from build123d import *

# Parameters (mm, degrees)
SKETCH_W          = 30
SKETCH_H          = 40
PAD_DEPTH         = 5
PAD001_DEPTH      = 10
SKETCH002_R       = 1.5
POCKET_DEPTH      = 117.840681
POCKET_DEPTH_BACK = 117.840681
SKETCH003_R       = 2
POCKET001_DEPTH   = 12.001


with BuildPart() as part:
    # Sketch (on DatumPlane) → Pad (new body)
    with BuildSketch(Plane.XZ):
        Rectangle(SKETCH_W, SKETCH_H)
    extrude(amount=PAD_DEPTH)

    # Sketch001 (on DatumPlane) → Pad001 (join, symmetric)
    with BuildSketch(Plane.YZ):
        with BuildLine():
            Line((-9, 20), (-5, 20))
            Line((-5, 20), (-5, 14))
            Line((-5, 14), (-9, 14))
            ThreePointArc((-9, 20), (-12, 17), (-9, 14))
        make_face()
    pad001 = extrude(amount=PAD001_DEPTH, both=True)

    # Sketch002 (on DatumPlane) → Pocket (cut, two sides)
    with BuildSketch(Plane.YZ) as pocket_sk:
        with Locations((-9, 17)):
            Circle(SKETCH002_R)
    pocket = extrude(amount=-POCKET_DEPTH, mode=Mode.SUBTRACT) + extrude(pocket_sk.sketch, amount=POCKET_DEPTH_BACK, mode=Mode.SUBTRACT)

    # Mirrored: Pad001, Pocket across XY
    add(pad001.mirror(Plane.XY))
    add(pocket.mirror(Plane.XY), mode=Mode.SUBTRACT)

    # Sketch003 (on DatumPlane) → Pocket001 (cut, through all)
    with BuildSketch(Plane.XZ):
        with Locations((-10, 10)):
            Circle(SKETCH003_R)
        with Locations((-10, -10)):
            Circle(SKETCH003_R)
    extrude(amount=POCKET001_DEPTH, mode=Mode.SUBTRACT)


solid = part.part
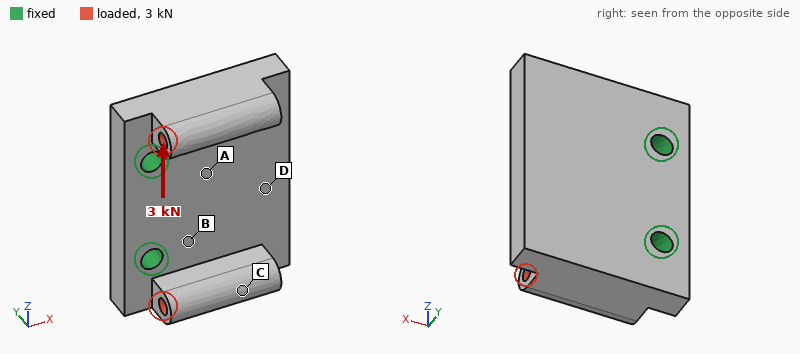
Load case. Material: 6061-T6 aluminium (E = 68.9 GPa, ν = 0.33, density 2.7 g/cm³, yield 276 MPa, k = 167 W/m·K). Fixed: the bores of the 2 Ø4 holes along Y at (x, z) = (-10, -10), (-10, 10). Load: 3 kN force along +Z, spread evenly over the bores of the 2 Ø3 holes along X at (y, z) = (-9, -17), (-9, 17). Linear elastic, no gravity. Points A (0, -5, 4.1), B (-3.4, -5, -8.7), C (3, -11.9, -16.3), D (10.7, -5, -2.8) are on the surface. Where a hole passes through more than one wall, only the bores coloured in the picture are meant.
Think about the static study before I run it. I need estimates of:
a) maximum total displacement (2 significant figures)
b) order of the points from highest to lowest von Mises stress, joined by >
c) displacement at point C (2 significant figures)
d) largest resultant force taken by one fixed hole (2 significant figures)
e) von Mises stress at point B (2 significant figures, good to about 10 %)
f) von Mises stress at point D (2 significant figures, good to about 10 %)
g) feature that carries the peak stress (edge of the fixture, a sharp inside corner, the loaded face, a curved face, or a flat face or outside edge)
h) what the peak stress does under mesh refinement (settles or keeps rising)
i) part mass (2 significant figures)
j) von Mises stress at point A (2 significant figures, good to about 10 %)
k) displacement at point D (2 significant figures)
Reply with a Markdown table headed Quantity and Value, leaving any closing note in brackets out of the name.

| Quantity | Value |
|---|---|
| maximum total displacement | 84 µm |
| order of the points from highest to lowest von Mises stress, joined by > | B > A > D > C |
| displacement at point C | 69 µm |
| largest resultant force taken by one fixed hole | 2.0 kN |
| von Mises stress at point B | 75 MPa |
| von Mises stress at point D | 27 MPa |
| feature that carries the peak stress | edge of the fixture |
| what the peak stress does under mesh refinement | keeps rising |
| part mass | 19 g |
| von Mises stress at point A | 52 MPa |
| displacement at point D | 18 µm |
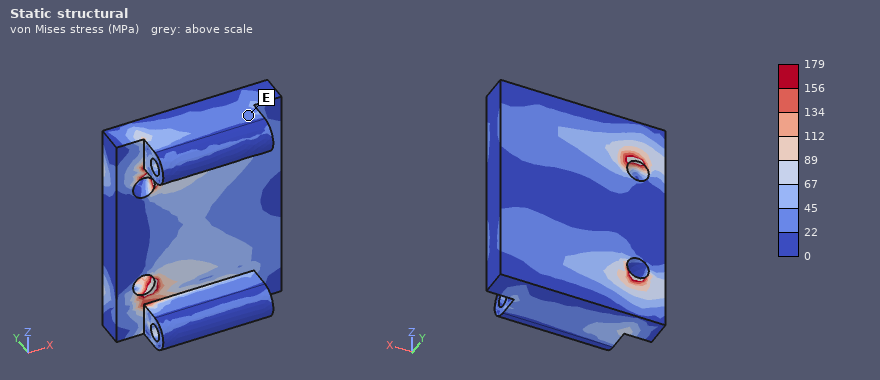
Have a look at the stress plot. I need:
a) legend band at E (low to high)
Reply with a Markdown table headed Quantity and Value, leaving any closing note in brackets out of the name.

| Quantity | Value |
|---|---|
| legend band at E | 22 to 45 MPa |
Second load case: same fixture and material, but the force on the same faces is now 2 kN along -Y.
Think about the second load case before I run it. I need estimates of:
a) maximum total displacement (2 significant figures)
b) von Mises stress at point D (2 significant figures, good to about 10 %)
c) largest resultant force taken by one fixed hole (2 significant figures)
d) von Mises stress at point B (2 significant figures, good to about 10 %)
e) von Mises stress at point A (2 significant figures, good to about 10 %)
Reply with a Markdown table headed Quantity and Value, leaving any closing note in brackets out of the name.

| Quantity | Value |
|---|---|
| maximum total displacement | 0.10 mm |
| von Mises stress at point D | 30 MPa |
| largest resultant force taken by one fixed hole | 1.0 kN |
| von Mises stress at point B | 58 MPa |
| von Mises stress at point A | 34 MPa |
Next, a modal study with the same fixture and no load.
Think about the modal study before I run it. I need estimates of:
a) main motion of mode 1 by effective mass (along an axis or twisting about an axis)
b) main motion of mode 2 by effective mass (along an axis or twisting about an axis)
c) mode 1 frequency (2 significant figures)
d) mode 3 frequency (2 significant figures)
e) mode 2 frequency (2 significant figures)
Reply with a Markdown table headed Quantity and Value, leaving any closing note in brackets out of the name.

| Quantity | Value |
|---|---|
| main motion of mode 1 by effective mass | along Y |
| main motion of mode 2 by effective mass | twisting about X |
| mode 1 frequency | 6400 Hz |
| mode 3 frequency | 17 kHz |
| mode 2 frequency | 8900 Hz |
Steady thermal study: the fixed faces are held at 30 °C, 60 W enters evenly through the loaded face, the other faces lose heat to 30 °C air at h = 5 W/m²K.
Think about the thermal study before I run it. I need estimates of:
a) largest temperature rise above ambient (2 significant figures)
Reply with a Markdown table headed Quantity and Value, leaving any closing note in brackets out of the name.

| Quantity | Value |
|---|---|
| largest temperature rise above ambient | 32 K |
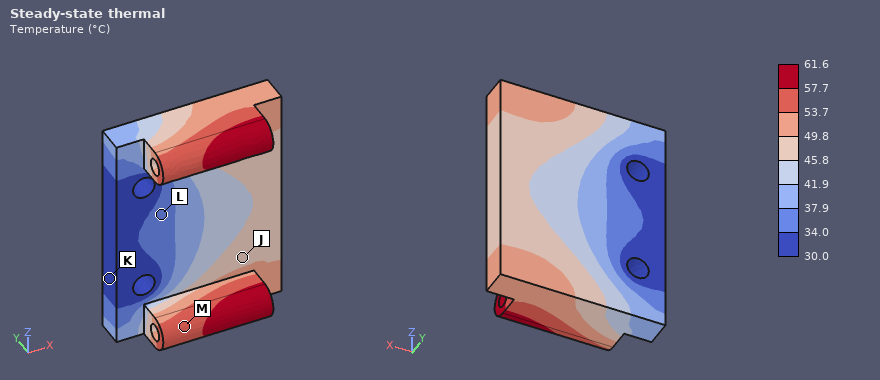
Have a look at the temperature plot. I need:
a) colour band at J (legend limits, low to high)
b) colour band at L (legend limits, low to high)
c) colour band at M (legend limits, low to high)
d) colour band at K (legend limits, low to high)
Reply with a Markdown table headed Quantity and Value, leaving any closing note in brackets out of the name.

| Quantity | Value |
|---|---|
| colour band at J | 45.8 to 49.8 °C |
| colour band at L | 34.0 to 37.9 °C |
| colour band at M | 53.7 to 57.7 °C |
| colour band at K | 30.0 to 34.0 °C |
